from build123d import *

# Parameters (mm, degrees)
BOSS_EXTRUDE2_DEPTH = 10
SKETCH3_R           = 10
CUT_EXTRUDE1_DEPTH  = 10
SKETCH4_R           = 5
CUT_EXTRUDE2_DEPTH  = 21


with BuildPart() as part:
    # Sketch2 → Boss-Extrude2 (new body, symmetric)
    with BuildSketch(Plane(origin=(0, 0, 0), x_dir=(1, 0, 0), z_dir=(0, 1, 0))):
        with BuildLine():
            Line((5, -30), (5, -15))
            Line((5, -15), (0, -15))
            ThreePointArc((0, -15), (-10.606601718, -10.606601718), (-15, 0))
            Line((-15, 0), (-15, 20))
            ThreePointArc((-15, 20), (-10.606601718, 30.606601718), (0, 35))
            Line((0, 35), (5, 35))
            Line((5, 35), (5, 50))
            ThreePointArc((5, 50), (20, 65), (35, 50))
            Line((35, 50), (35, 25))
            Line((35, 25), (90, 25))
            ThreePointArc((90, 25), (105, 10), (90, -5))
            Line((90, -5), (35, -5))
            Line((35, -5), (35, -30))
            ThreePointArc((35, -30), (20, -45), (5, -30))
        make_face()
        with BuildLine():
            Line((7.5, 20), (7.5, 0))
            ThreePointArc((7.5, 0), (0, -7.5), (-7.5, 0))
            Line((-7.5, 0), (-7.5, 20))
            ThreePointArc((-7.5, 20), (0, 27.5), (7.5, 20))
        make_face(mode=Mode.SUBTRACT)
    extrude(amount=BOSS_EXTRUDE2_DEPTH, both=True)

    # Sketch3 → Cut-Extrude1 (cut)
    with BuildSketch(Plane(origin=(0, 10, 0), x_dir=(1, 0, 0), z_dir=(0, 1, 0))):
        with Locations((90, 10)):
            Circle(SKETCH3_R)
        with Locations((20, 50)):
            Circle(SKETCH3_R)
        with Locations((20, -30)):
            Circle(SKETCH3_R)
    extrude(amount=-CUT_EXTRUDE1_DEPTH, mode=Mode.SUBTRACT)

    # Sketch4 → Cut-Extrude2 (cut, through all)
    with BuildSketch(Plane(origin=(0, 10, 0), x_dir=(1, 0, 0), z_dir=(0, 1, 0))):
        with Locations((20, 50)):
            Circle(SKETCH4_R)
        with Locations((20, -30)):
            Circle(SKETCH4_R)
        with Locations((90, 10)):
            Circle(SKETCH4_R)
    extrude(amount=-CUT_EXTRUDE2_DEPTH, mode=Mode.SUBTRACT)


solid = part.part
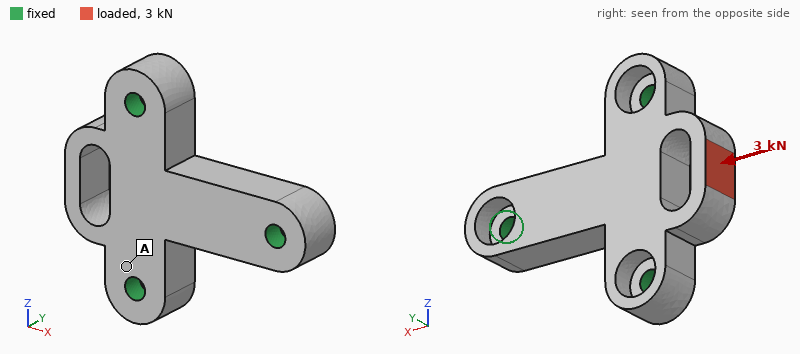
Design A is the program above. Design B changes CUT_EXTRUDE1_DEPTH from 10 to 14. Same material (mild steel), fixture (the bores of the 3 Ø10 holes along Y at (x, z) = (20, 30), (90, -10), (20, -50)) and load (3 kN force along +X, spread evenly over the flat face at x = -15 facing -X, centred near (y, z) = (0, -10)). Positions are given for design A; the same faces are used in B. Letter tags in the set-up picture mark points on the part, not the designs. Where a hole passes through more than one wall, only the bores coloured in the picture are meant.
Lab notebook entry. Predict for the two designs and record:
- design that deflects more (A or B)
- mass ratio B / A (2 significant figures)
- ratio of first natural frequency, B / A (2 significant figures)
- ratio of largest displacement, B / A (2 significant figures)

B
0.97
0.87
1.1
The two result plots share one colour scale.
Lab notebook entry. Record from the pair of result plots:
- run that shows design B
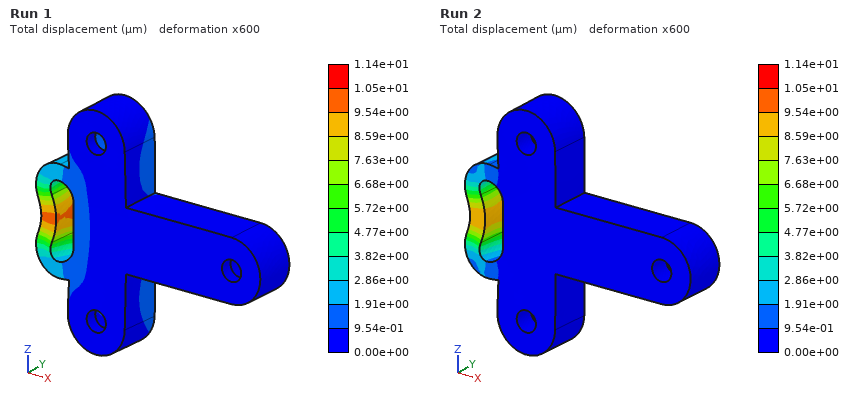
Run 1
